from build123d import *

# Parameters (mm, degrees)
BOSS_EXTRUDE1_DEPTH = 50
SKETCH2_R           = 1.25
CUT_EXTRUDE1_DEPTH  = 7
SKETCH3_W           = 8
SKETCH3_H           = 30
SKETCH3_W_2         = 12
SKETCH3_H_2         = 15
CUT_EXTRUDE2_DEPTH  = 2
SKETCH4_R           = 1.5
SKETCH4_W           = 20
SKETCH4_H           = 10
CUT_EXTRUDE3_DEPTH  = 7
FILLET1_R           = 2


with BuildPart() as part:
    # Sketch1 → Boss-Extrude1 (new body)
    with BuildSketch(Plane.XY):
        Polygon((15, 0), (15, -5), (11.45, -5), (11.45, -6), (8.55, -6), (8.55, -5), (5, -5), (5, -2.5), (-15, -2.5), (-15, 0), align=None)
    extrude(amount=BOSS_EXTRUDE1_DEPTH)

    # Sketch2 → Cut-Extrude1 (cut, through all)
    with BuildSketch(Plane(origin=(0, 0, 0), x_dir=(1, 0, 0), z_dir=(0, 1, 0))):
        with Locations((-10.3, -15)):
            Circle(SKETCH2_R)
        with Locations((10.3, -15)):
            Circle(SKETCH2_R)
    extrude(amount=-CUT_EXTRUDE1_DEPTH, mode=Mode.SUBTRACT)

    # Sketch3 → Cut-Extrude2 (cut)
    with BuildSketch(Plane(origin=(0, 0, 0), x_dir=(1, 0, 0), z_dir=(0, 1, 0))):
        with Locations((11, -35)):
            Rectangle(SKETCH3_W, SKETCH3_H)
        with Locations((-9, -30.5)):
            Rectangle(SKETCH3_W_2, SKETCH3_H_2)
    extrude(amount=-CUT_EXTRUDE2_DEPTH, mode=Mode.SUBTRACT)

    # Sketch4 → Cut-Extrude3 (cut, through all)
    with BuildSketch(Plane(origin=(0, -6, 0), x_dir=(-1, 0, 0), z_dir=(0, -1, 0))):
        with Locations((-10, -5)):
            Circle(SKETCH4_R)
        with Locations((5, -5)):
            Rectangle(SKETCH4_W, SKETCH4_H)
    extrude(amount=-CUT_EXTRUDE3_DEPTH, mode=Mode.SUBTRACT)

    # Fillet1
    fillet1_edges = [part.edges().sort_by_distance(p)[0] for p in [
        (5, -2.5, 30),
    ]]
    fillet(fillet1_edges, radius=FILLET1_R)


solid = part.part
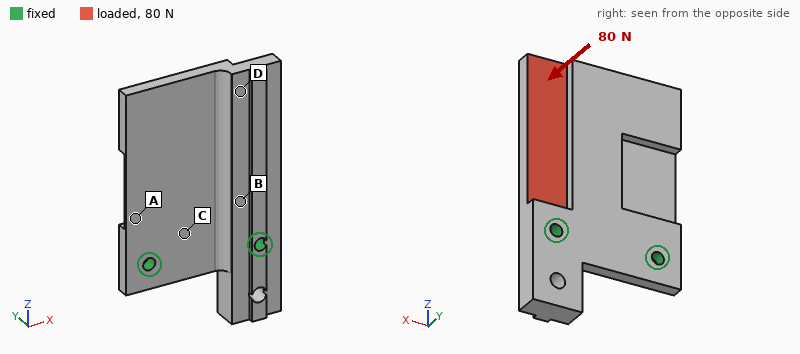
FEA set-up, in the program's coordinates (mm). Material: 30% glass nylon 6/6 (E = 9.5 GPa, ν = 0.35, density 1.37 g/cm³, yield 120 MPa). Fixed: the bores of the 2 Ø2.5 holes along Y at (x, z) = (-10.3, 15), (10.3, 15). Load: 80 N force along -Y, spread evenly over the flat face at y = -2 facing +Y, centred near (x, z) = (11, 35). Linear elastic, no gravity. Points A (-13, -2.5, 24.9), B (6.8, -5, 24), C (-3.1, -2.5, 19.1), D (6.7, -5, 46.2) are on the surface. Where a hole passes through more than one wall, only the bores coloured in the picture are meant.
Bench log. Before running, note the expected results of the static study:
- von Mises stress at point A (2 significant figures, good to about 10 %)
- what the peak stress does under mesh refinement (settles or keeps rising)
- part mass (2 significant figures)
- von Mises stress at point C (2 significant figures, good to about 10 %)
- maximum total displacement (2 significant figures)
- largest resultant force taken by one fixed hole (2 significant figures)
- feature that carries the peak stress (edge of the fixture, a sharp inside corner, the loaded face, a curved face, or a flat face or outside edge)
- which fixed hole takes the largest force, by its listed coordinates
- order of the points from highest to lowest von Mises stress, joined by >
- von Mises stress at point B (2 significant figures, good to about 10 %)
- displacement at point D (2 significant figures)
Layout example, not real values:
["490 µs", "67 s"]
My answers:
["12 MPa", "keeps rising", "5.1 g", "6.1 MPa", "0.58 mm", "88 N", "edge of the fixture", "(10.3, 15)", "B > A > C > D", "22 MPa", "0.45 mm"]
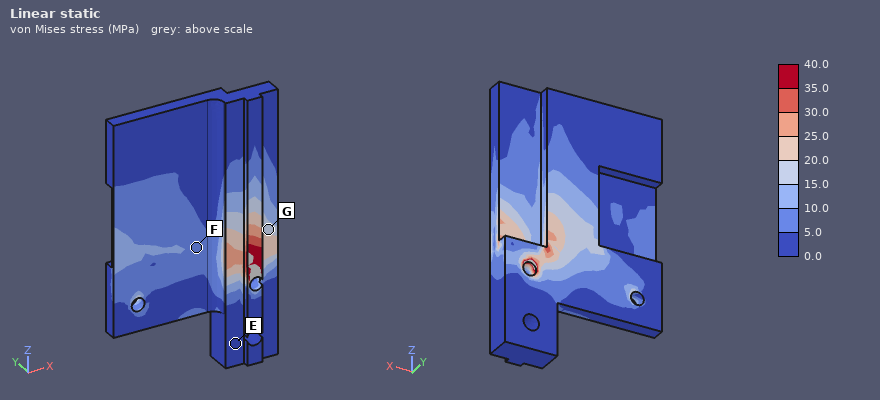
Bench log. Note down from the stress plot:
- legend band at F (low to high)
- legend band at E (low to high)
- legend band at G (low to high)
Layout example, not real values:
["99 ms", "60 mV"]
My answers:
["5.0 to 10.0 MPa", "0.0 to 5.0 MPa", "15.0 to 20.0 MPa"]
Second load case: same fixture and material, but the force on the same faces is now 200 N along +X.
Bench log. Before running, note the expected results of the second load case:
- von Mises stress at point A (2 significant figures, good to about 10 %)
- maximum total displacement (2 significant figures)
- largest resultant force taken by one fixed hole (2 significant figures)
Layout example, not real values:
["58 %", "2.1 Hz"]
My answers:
["20 MPa", "0.15 mm", "210 N"]
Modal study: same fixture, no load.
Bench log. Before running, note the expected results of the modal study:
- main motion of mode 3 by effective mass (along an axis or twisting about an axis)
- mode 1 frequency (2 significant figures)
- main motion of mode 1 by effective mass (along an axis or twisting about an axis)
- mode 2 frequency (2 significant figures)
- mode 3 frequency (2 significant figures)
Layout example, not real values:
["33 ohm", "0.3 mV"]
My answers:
["along X", "1200 Hz", "along Y", "2300 Hz", "5400 Hz"]
